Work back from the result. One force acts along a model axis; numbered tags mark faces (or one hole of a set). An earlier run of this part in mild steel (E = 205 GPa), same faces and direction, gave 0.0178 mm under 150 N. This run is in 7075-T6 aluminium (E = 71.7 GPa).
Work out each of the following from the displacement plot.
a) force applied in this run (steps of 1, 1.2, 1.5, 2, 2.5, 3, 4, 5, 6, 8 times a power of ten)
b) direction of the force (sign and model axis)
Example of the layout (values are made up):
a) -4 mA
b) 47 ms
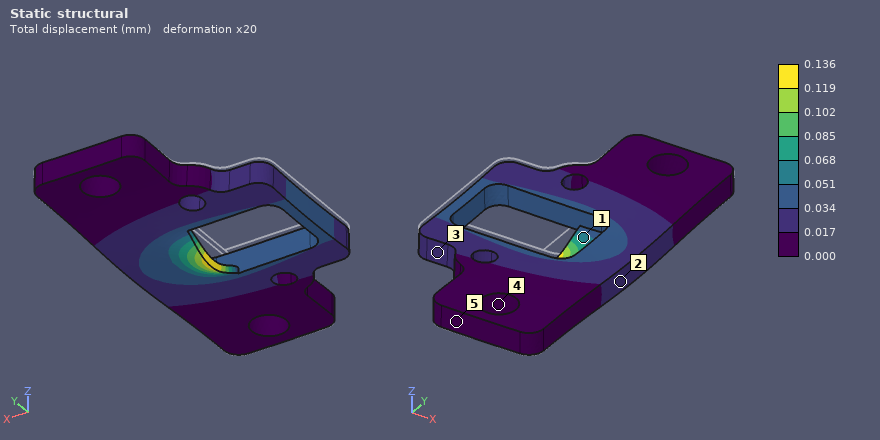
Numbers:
a) 400 N
b) -Z
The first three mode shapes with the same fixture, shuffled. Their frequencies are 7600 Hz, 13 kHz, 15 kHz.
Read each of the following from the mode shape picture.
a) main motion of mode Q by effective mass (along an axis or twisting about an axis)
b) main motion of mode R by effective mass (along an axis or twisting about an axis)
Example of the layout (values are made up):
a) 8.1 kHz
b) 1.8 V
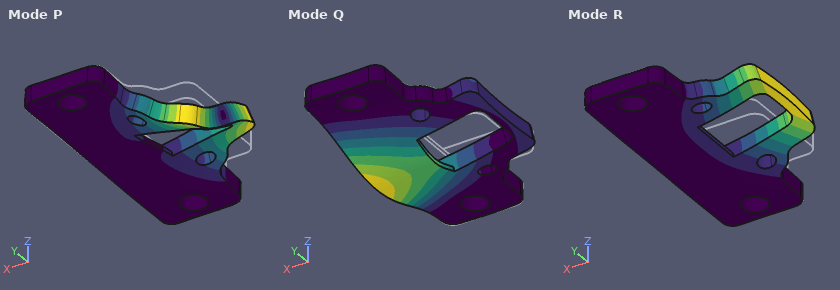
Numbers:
a) along Z
b) along Z
